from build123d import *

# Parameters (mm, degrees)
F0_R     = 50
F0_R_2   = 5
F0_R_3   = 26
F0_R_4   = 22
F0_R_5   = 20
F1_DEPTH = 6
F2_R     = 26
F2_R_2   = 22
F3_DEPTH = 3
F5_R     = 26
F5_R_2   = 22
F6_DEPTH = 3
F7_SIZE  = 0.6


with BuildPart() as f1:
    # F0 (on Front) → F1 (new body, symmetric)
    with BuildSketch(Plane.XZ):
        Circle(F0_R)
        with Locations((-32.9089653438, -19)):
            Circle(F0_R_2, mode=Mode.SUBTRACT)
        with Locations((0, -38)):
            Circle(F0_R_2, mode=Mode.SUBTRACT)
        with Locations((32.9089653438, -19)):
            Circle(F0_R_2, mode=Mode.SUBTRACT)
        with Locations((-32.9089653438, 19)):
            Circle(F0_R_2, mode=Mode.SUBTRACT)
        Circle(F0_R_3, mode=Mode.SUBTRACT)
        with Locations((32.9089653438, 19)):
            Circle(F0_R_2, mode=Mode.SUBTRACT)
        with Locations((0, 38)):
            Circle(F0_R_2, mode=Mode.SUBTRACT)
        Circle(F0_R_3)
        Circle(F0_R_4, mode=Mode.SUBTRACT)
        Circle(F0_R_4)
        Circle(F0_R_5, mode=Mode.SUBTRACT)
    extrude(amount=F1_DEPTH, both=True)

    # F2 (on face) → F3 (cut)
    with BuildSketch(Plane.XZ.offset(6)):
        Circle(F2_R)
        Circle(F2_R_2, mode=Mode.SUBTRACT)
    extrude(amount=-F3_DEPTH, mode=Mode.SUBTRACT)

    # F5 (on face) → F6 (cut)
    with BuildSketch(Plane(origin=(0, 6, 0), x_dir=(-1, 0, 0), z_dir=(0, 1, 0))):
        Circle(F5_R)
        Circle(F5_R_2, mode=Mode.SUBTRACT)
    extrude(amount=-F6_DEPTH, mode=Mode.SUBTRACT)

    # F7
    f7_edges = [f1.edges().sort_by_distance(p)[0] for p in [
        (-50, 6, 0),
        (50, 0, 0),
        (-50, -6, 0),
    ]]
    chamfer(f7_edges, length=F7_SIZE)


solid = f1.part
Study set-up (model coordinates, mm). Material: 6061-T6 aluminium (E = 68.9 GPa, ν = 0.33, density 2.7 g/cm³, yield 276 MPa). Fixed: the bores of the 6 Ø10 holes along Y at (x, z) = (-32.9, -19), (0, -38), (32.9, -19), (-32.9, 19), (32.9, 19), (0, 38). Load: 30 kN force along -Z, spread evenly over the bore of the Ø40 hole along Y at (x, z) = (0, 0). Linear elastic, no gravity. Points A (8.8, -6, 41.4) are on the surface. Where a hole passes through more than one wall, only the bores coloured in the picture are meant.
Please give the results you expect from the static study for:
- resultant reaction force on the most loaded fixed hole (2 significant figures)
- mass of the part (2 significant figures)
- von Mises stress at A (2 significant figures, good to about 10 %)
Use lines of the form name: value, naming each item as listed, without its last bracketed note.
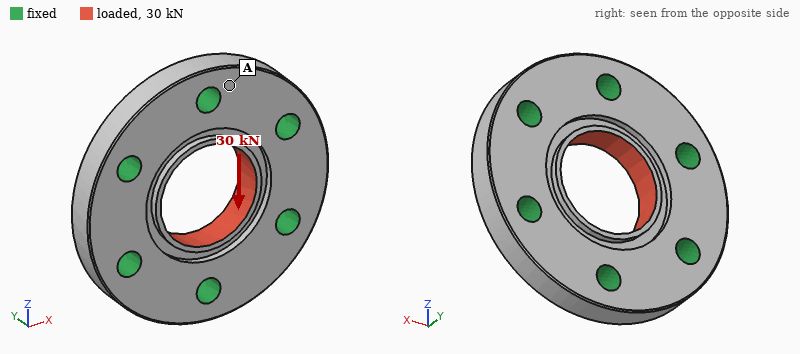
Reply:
resultant reaction force on the most loaded fixed hole: 6.9 kN
mass of the part: 190 g
von Mises stress at A: 13 MPa
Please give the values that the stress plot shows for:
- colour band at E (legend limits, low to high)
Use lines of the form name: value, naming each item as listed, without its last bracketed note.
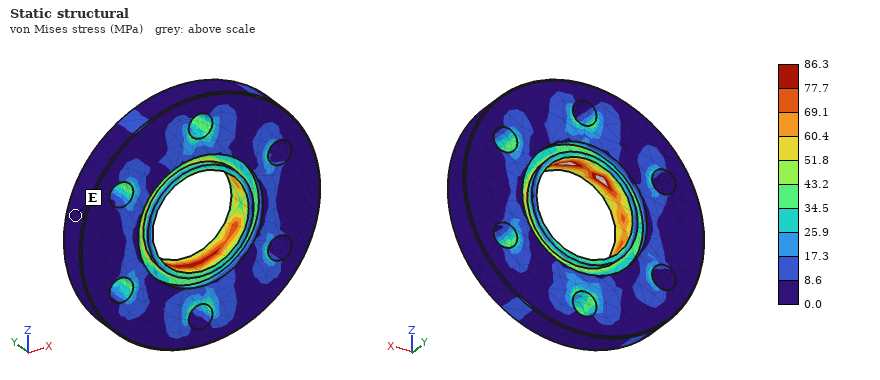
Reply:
colour band at E: 0.0 to 8.6 MPa
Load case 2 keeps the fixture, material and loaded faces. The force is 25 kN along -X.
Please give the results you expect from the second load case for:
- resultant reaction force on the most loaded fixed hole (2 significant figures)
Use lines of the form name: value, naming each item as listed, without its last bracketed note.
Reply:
resultant reaction force on the most loaded fixed hole: 5.2 kN
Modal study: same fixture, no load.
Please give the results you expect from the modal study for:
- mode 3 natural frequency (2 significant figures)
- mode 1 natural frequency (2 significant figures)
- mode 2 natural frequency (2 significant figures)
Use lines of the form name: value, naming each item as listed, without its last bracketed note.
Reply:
mode 3 natural frequency: 27 kHz
mode 1 natural frequency: 27 kHz
mode 2 natural frequency: 27 kHz
